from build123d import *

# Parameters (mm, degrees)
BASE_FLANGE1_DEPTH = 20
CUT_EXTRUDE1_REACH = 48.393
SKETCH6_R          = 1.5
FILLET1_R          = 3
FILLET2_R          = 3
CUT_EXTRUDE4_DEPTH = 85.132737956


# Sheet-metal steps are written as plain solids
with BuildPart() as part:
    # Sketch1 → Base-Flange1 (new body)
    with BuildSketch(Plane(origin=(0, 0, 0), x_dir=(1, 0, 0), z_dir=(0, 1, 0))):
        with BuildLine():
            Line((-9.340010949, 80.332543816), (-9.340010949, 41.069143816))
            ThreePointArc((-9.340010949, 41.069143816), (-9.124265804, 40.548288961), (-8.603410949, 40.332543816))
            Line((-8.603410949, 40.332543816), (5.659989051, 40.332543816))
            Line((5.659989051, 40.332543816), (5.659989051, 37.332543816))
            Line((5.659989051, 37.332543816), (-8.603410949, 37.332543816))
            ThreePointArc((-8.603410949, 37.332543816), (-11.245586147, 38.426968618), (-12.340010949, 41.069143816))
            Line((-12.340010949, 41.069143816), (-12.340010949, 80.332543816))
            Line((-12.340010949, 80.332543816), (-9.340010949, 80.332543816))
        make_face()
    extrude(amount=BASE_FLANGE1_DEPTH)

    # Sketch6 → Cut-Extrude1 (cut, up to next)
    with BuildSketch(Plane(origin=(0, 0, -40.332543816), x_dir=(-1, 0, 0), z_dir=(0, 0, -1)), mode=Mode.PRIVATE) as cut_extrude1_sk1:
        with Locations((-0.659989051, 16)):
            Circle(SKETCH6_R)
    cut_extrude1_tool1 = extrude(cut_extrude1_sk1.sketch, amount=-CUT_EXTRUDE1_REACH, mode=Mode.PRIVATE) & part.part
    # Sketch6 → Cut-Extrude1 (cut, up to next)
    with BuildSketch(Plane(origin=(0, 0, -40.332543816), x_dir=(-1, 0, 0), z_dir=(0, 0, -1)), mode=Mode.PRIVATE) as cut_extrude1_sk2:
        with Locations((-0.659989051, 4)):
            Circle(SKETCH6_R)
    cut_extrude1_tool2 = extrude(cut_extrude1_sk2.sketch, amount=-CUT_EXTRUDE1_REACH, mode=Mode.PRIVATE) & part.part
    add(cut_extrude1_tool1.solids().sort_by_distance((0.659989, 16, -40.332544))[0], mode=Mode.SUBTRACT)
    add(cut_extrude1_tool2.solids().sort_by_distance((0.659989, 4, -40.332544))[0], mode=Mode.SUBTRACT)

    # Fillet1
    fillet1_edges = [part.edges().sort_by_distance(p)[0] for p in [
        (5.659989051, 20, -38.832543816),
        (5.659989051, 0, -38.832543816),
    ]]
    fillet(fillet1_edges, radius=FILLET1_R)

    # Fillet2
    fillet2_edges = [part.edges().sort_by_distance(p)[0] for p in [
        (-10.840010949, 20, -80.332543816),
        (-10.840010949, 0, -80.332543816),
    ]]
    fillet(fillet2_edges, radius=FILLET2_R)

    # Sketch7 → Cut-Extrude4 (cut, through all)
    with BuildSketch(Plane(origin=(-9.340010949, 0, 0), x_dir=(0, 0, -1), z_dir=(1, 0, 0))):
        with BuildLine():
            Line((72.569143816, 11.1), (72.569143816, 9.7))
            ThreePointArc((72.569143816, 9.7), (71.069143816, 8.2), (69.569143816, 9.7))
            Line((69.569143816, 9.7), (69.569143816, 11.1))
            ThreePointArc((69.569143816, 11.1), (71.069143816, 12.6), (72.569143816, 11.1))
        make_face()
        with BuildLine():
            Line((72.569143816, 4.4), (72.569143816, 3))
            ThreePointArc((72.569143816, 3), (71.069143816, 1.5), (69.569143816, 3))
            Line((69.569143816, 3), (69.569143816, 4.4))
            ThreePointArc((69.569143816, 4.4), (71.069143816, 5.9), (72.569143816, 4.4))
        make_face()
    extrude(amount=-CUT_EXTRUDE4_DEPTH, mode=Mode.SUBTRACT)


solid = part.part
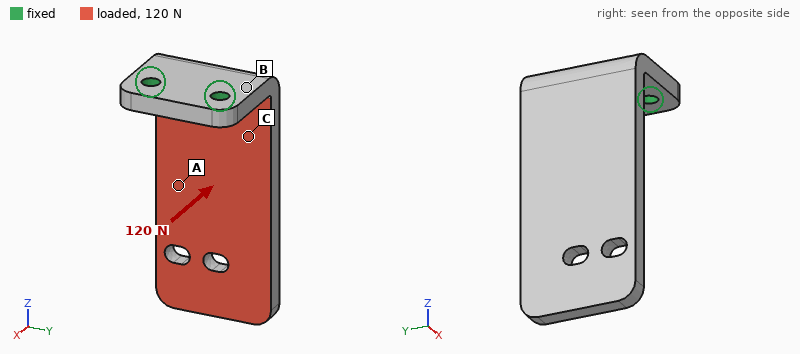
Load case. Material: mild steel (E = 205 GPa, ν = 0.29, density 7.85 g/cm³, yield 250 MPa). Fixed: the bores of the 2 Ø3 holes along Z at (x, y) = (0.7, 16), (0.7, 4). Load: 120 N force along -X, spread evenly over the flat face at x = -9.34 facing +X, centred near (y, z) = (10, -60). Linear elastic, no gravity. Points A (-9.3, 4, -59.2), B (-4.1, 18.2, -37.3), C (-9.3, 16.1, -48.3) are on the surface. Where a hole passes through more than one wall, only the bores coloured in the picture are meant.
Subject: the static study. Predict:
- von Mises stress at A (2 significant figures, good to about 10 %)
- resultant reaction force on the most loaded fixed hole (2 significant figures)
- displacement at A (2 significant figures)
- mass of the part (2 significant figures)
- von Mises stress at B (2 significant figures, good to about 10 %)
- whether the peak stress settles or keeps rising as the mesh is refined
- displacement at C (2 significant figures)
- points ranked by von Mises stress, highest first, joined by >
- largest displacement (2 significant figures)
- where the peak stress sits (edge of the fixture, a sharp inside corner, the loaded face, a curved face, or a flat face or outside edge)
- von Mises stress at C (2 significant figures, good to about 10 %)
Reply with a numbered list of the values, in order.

1. 22 MPa
2. 66 N
3. 0.095 mm
4. 26 g
5. 85 MPa
6. keeps rising
7. 0.037 mm
8. B > C > A
9. 0.23 mm
10. edge of the fixture
11. 49 MPa
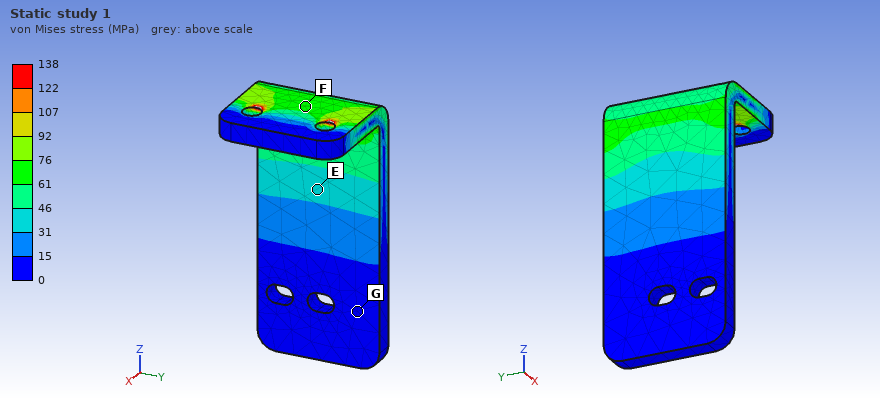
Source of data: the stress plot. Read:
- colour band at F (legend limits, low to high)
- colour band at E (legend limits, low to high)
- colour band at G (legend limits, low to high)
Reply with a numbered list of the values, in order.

1. 61 to 76 MPa
2. 31 to 46 MPa
3. 0 to 15 MPa
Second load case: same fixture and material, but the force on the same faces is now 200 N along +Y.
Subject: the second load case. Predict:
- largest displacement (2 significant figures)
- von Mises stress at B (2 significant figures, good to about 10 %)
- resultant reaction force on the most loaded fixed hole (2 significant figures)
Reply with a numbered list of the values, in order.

1. 78 µm
2. 70 MPa
3. 340 N
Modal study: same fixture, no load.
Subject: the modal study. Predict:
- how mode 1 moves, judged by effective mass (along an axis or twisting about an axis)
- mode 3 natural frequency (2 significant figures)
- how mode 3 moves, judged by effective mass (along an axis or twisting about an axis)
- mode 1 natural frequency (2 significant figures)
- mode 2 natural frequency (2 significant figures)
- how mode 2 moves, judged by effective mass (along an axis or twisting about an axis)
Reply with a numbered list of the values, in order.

1. along X
2. 5600 Hz
3. along Z
4. 1100 Hz
5. 2300 Hz
6. along Y
